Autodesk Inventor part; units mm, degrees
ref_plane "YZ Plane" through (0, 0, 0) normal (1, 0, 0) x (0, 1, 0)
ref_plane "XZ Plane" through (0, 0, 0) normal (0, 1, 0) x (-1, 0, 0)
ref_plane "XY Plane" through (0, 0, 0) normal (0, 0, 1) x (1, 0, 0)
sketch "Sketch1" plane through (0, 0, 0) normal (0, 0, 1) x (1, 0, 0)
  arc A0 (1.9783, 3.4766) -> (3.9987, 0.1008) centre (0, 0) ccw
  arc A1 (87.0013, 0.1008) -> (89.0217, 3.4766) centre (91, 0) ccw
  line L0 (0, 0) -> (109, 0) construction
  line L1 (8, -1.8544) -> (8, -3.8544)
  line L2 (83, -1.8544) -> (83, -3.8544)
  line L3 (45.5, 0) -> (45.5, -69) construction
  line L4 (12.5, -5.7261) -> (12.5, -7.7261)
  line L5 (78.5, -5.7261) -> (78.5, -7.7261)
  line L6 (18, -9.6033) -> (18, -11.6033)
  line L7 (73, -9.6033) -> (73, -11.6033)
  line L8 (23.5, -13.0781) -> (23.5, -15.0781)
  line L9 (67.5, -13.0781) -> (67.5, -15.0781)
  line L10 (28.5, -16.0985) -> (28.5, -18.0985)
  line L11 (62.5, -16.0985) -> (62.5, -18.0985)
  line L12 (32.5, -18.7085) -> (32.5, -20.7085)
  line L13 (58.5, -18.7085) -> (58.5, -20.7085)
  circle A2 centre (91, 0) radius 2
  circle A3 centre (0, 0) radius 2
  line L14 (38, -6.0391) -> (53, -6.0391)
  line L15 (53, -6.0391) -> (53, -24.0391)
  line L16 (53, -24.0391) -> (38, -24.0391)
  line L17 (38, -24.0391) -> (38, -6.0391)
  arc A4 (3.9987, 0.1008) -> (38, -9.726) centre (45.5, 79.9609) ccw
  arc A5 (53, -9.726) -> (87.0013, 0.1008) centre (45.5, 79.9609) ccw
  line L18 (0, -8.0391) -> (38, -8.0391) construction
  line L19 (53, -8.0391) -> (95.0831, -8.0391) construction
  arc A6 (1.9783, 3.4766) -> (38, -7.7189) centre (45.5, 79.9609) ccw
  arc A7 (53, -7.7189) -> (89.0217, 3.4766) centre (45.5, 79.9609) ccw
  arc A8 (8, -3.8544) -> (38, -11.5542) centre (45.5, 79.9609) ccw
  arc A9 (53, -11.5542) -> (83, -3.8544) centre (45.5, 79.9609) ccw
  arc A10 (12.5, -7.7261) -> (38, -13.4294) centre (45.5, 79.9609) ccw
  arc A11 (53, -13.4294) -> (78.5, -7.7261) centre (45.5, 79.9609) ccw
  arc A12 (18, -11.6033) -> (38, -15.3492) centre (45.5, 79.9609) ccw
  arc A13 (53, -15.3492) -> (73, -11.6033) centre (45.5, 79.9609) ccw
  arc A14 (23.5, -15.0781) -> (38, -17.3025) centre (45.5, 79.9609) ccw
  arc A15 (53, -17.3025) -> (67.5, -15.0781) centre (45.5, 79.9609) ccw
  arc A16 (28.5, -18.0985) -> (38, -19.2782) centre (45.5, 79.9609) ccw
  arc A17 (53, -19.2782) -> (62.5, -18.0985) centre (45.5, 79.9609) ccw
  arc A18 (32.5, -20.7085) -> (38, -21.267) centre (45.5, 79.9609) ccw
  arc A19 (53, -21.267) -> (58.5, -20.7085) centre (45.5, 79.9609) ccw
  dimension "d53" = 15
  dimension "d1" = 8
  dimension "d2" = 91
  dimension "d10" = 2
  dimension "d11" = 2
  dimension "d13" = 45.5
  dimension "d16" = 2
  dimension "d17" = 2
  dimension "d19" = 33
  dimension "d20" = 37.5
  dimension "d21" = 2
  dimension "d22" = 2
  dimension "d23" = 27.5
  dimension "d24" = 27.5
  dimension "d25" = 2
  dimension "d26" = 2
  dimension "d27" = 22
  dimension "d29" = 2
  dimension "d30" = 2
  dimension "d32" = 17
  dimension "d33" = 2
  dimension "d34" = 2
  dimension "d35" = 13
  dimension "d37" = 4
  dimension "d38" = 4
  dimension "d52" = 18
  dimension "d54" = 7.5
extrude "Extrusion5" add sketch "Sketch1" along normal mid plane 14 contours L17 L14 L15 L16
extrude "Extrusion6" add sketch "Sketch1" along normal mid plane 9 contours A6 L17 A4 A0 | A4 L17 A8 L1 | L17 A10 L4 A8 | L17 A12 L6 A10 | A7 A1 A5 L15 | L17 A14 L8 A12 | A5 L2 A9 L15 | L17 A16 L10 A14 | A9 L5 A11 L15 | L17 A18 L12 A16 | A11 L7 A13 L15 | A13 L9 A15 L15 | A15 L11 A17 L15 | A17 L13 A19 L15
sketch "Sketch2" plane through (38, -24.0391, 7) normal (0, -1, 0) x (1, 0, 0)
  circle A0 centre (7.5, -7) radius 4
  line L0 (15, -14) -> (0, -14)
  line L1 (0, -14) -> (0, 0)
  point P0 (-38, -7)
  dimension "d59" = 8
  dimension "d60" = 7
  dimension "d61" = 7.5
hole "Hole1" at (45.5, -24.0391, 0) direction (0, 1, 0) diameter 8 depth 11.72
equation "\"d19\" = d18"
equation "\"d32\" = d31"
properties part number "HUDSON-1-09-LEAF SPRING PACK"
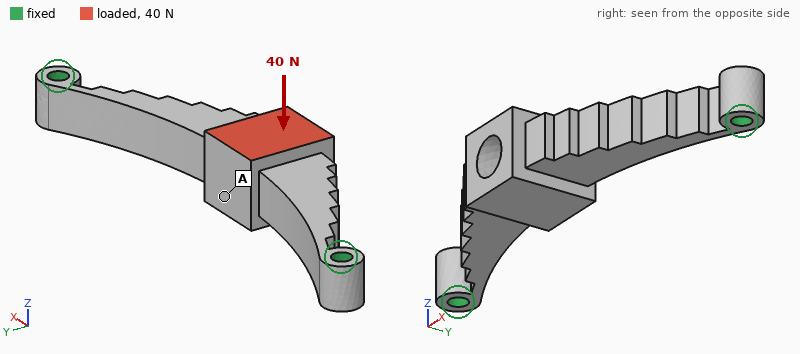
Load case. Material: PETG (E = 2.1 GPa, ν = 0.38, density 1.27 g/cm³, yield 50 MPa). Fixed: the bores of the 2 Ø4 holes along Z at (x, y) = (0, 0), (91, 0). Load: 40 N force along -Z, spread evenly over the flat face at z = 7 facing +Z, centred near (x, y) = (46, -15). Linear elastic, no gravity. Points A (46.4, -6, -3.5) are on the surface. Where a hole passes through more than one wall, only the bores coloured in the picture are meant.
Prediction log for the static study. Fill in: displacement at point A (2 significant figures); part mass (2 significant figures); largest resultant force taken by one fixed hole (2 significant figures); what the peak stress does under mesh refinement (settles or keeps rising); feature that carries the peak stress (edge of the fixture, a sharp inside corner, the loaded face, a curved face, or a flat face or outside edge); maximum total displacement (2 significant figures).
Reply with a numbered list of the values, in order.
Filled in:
1. 0.32 mm
2. 11 g
3. 20 N
4. keeps rising
5. a sharp inside corner
6. 1.1 mm
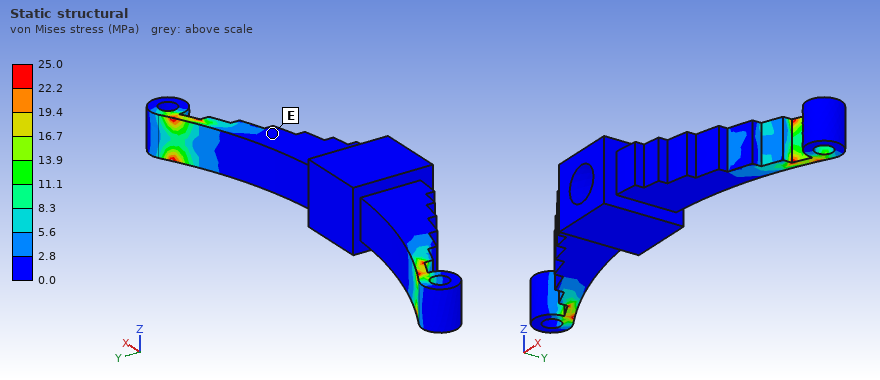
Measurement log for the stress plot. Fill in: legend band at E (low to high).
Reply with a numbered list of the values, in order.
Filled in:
1. 0.0 to 2.8 MPa
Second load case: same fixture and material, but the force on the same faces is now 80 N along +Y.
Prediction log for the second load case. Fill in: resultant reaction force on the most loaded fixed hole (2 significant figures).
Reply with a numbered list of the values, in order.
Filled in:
1. 79 N
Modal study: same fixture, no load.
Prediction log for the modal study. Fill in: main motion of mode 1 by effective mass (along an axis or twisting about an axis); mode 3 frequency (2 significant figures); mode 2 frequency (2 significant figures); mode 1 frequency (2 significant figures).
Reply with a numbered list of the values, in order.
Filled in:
1. along Z
2. 1600 Hz
3. 1600 Hz
4. 440 Hz
